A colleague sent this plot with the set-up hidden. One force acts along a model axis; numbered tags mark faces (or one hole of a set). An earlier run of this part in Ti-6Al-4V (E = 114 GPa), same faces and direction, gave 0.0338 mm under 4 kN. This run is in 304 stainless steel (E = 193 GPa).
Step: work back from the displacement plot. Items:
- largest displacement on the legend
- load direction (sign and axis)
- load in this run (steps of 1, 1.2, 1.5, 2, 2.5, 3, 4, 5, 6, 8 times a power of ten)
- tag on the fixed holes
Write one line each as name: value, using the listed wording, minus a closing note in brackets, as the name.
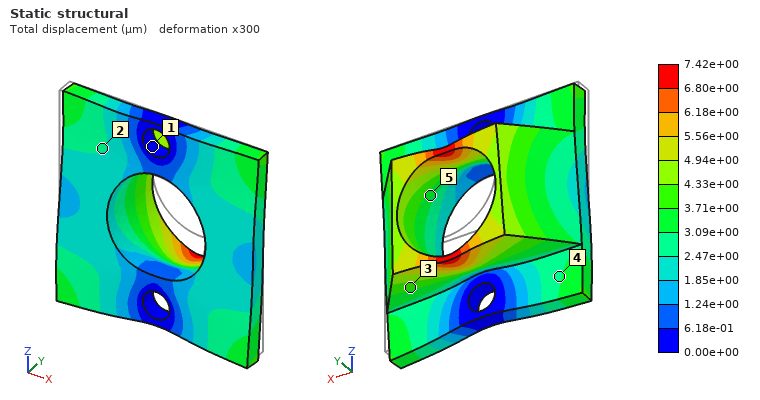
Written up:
largest displacement on the legend: 7.42e+00 µm
load direction: -Z
load in this run: 1.5 kN
tag on the fixed holes: 1
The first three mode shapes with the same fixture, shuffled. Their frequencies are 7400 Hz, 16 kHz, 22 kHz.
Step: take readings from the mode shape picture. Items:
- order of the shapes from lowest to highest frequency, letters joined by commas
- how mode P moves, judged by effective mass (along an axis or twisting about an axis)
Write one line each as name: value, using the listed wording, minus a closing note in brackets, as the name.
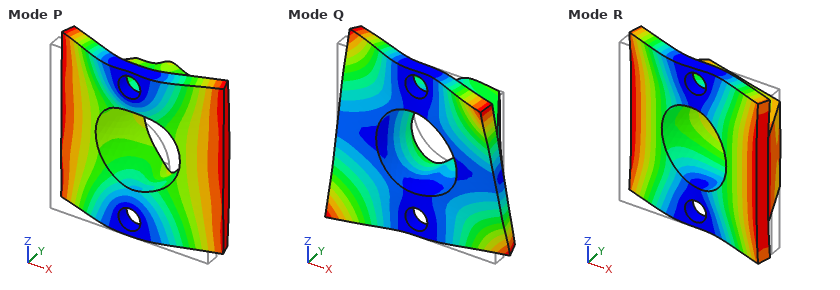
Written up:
order of the shapes from lowest to highest frequency, letters joined by commas: R, P, Q
how mode P moves, judged by effective mass: along Y
